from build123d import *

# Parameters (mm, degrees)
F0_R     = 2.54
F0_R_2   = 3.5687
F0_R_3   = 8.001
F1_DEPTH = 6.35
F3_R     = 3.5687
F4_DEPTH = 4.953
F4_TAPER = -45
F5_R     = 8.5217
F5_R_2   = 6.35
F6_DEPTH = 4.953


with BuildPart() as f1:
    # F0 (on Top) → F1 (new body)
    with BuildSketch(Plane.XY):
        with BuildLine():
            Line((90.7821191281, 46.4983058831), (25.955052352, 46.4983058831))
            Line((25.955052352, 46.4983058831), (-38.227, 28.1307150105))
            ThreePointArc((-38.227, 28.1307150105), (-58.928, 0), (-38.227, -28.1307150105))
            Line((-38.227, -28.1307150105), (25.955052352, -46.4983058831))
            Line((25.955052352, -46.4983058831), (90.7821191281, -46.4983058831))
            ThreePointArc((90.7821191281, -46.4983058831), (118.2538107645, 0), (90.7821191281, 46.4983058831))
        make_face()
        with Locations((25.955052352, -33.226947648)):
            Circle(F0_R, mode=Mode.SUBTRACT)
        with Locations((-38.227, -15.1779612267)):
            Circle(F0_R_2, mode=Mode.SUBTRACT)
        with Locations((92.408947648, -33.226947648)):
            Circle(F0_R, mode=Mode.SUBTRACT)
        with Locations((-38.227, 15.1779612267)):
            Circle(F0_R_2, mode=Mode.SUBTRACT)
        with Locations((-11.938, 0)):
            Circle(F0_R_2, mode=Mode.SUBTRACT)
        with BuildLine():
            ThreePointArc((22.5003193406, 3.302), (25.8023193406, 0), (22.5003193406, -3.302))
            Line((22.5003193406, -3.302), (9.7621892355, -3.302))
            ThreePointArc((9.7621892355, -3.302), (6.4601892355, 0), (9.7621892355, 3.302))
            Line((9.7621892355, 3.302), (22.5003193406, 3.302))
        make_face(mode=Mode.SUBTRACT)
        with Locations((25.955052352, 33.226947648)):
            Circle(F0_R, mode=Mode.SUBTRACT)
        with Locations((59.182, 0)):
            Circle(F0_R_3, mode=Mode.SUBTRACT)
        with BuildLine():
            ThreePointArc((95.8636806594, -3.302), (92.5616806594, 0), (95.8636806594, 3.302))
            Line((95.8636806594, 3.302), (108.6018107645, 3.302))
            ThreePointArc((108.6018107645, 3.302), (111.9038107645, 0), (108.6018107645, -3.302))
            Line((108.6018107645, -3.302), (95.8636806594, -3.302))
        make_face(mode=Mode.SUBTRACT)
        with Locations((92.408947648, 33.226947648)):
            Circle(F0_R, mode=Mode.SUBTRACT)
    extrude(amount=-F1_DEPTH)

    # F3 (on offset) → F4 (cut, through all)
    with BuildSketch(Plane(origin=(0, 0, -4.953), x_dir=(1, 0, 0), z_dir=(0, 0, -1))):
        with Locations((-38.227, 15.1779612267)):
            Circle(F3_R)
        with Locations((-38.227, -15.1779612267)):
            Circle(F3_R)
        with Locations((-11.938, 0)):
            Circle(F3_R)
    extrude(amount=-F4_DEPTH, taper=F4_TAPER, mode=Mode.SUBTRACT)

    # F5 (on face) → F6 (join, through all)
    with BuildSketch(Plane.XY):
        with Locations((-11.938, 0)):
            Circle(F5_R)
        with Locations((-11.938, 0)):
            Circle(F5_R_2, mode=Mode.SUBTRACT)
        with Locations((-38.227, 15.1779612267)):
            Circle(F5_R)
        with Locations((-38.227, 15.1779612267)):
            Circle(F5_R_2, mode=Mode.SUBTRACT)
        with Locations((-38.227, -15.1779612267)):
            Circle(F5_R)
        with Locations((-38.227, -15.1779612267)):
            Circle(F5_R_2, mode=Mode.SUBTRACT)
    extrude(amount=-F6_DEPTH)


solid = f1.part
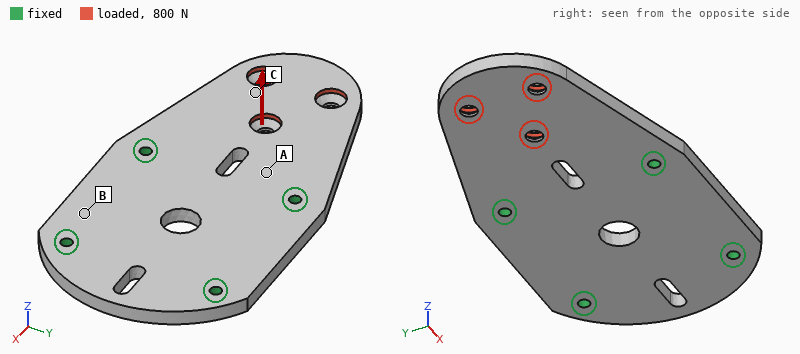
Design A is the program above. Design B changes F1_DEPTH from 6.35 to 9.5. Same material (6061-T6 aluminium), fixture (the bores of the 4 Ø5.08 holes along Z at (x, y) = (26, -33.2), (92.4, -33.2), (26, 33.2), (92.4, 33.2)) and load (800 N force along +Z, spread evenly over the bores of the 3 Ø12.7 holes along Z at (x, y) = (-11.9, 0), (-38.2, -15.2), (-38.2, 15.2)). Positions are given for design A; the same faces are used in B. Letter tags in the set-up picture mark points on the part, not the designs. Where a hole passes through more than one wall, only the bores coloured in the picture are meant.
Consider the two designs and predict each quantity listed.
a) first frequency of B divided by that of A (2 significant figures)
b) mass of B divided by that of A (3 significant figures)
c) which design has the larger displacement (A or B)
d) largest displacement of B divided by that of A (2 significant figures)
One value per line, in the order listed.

1.4
1.50
A
0.31
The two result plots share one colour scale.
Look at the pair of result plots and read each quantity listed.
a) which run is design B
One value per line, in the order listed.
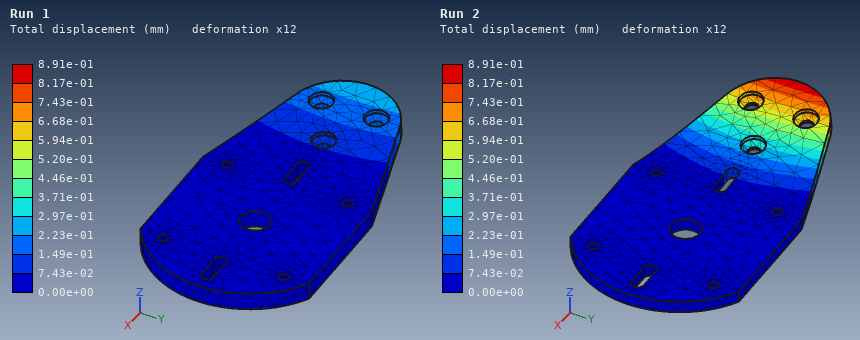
Run 1
